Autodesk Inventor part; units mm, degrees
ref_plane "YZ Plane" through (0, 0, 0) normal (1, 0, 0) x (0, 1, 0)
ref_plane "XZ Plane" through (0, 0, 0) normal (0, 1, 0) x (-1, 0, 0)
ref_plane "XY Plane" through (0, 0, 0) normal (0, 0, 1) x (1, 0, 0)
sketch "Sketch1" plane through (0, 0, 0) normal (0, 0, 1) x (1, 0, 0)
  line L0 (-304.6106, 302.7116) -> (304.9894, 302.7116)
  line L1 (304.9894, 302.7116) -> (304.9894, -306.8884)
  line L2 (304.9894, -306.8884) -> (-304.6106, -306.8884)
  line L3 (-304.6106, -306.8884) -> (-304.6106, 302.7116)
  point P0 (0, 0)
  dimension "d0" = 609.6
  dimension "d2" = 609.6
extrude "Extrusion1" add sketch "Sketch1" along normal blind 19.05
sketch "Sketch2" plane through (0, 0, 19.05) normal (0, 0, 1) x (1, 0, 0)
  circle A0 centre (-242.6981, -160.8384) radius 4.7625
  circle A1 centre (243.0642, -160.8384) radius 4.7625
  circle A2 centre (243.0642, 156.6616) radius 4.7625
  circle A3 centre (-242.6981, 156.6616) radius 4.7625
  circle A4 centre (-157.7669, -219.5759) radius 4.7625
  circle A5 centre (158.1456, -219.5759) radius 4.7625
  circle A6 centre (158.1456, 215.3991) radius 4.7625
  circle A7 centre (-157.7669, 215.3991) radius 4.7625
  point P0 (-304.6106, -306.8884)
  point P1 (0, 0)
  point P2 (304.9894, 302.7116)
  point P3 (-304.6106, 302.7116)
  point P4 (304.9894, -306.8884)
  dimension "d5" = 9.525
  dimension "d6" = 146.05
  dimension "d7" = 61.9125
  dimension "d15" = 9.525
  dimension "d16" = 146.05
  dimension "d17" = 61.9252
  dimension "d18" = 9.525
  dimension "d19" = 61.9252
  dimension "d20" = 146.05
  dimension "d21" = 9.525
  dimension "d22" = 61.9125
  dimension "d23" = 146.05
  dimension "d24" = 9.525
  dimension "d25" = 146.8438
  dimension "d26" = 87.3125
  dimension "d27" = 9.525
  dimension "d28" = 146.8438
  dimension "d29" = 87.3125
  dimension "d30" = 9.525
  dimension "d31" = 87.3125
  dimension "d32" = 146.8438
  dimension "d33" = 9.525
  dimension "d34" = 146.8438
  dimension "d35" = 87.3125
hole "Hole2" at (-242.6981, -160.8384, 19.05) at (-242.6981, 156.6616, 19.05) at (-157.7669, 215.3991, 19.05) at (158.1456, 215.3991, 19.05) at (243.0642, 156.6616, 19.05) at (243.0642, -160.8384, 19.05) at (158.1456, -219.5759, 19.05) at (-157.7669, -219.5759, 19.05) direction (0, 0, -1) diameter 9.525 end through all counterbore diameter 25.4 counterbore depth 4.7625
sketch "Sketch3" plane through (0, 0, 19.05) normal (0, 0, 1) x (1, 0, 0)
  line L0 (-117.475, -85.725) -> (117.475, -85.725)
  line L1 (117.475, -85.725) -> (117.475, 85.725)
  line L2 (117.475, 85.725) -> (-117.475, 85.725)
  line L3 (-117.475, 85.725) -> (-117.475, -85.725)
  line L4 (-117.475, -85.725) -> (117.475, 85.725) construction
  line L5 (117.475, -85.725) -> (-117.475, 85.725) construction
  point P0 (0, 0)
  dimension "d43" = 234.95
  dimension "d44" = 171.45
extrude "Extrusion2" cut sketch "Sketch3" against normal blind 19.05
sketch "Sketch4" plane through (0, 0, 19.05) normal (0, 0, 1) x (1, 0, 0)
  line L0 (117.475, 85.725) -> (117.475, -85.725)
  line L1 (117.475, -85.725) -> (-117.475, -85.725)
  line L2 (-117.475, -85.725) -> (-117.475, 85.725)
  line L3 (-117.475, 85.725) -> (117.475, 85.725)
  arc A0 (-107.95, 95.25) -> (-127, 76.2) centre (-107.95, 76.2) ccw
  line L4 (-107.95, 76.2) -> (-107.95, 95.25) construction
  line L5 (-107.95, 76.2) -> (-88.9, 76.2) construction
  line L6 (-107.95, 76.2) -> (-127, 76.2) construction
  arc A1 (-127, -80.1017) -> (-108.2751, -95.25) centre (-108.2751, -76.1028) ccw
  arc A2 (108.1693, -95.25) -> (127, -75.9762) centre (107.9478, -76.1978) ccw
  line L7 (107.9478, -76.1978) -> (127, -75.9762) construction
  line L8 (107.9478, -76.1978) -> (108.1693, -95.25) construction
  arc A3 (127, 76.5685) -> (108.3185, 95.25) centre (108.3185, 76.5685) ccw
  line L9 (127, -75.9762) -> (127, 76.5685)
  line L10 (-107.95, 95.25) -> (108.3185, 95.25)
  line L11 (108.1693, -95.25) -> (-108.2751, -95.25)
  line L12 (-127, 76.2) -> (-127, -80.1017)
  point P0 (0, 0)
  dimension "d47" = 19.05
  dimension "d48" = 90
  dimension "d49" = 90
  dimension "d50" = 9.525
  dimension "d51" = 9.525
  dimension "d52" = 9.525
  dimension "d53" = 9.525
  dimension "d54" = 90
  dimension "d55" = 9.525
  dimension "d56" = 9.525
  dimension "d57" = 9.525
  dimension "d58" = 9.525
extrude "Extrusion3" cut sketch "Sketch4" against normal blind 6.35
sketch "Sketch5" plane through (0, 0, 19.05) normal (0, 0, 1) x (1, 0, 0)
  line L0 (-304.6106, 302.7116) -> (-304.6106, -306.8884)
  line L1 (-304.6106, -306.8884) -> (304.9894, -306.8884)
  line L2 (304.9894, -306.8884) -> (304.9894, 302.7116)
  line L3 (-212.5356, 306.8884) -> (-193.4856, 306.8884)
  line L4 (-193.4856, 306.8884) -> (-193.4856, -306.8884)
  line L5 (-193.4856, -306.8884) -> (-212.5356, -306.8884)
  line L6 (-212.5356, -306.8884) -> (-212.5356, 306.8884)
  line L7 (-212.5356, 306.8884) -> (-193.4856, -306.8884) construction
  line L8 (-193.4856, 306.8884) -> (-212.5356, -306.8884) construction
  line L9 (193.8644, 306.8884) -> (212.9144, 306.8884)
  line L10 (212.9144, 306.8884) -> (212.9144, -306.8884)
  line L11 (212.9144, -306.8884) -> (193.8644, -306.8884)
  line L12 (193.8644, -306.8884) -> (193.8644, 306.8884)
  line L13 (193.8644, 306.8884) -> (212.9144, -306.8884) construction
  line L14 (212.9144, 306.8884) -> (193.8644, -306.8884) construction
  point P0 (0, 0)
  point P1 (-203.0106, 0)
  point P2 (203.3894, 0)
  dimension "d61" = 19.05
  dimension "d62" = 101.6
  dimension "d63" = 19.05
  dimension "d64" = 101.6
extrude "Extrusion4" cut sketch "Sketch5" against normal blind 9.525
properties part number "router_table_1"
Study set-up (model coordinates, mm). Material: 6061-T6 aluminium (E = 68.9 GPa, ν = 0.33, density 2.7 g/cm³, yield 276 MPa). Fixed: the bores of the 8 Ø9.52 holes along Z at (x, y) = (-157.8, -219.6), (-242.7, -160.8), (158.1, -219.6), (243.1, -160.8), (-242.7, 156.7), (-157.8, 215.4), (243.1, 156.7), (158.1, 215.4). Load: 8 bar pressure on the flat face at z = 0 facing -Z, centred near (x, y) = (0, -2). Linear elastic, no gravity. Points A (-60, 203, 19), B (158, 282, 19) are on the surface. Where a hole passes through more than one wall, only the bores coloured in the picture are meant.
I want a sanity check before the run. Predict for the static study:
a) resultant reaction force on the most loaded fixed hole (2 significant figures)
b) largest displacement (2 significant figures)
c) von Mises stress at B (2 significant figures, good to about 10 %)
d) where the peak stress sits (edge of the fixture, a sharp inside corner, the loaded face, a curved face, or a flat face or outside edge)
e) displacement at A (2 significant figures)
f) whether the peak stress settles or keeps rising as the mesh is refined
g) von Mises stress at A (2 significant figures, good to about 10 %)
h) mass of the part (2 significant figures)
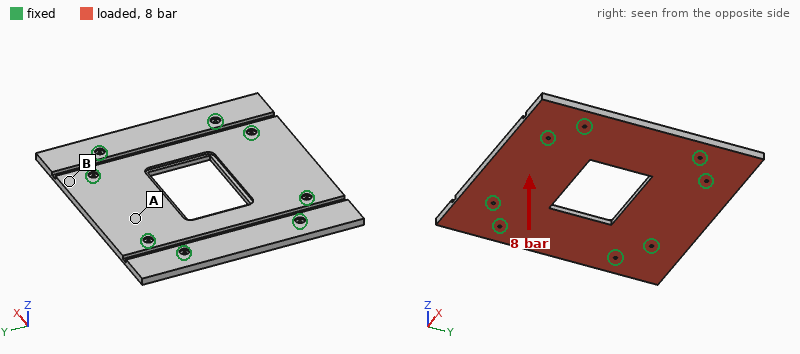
41 kN
2.7 mm
43 MPa
edge of the fixture
1.0 mm
keeps rising
84 MPa
16 kg
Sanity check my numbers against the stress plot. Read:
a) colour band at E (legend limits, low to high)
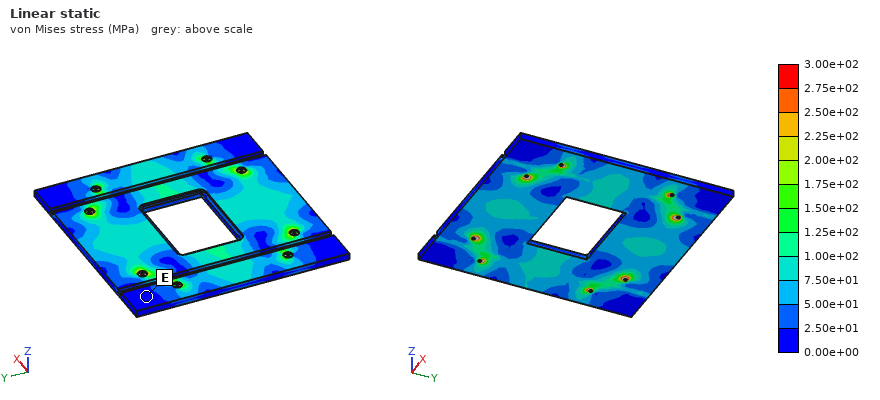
0.00e+00 to 2.50e+01 MPa
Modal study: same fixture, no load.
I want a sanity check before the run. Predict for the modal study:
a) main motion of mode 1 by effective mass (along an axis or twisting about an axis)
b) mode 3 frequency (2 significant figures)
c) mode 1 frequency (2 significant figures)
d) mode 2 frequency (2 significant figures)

along Z
670 Hz
470 Hz
660 Hz
